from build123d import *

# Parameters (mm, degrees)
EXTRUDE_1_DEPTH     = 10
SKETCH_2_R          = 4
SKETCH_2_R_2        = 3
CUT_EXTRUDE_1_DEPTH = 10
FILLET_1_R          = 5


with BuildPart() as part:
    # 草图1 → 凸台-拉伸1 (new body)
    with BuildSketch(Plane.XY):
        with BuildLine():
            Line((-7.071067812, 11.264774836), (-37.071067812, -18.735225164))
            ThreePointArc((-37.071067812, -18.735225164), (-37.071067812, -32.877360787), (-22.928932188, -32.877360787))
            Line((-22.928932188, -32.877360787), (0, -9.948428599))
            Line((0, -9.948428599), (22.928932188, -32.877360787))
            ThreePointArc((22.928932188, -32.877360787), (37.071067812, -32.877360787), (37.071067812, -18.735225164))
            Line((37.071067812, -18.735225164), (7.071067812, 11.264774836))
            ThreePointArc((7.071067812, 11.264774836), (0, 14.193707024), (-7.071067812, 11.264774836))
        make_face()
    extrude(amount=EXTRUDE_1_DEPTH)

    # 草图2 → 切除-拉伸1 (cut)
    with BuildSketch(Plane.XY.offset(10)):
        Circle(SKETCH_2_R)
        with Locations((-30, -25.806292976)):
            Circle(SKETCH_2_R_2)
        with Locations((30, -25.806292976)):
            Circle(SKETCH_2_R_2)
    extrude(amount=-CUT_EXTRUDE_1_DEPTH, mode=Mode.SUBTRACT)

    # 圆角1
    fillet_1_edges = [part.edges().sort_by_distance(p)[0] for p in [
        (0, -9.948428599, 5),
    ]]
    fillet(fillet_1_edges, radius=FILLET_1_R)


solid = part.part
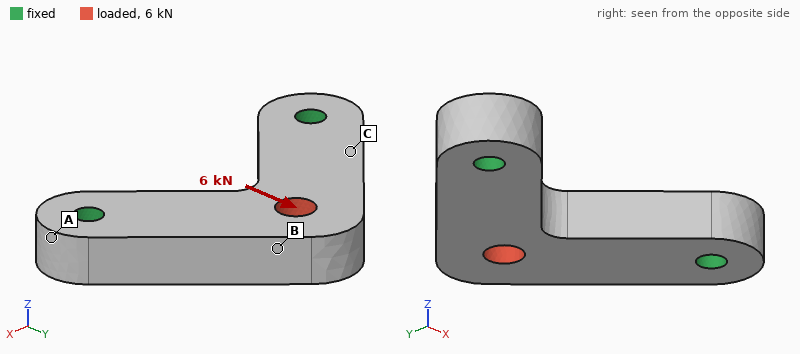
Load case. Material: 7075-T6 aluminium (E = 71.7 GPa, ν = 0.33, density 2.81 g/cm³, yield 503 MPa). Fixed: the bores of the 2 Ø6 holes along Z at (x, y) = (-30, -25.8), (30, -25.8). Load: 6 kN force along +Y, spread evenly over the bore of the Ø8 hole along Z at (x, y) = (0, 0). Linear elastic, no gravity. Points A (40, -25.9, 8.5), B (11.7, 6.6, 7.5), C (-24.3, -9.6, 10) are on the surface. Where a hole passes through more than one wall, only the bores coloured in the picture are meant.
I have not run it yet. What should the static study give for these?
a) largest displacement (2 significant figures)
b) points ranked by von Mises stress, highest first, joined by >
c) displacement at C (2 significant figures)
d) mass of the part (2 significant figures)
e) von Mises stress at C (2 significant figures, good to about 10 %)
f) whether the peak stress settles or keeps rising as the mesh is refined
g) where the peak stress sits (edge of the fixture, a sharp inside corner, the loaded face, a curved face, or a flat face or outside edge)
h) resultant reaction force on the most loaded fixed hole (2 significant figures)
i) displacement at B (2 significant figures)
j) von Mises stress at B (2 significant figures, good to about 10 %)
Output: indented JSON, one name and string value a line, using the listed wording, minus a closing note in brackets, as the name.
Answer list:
{
  "largest displacement": "18 µm",
  "points ranked by von Mises stress, highest first, joined by >": "B > C > A",
  "displacement at C": "4.7 µm",
  "mass of the part": "53 g",
  "von Mises stress at C": "17 MPa",
  "whether the peak stress settles or keeps rising as the mesh is refined": "keeps rising",
  "where the peak stress sits": "edge of the fixture",
  "resultant reaction force on the most loaded fixed hole": "3.9 kN",
  "displacement at B": "14 µm",
  "von Mises stress at B": "29 MPa"
}
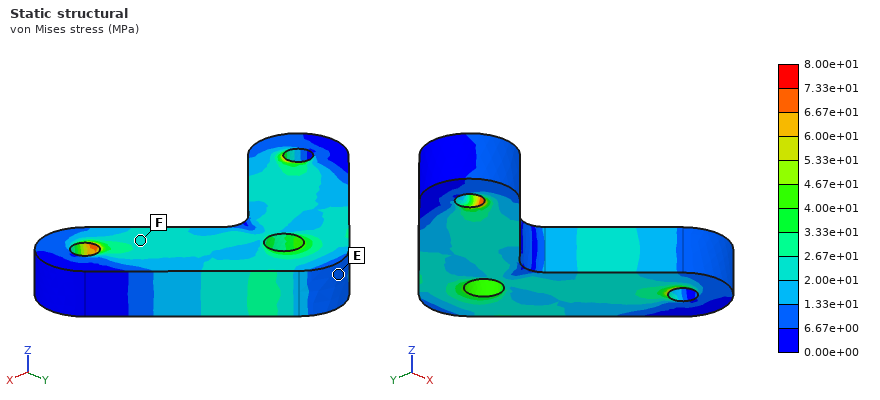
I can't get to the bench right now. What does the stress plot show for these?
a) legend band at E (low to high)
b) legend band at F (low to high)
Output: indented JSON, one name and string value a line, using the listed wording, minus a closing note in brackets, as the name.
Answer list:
{
  "legend band at E": "6.67e+00 to 1.33e+01 MPa",
  "legend band at F": "2.00e+01 to 2.67e+01 MPa"
}
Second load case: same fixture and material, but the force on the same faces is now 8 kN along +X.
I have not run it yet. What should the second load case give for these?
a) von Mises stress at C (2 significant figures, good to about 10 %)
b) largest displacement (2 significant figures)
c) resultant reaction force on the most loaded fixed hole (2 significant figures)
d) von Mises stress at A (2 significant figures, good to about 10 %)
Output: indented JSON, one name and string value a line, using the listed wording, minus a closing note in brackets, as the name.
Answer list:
{
  "von Mises stress at C": "25 MPa",
  "largest displacement": "27 µm",
  "resultant reaction force on the most loaded fixed hole": "5.1 kN",
  "von Mises stress at A": "11 MPa"
}
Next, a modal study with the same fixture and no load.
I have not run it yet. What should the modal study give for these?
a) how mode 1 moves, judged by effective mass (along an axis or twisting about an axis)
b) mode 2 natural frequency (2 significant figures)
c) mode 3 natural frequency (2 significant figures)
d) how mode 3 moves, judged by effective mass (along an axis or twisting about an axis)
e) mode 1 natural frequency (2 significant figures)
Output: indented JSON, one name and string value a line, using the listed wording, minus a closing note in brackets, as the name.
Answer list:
{
  "how mode 1 moves, judged by effective mass": "along Z",
  "mode 2 natural frequency": "16 kHz",
  "mode 3 natural frequency": "18 kHz",
  "how mode 3 moves, judged by effective mass": "along Z",
  "mode 1 natural frequency": "5100 Hz"
}
